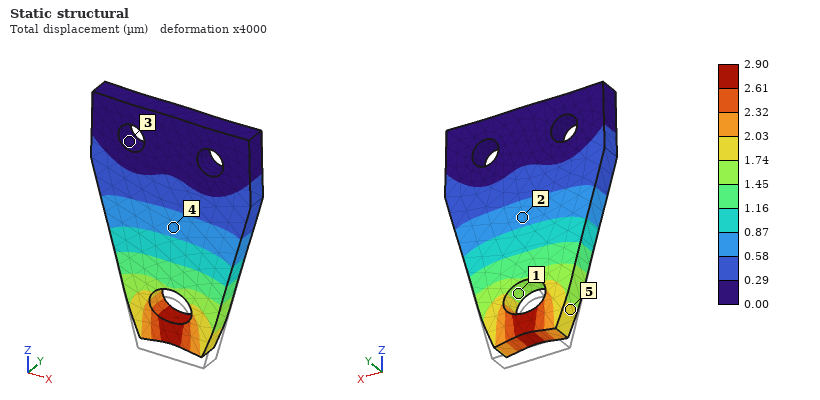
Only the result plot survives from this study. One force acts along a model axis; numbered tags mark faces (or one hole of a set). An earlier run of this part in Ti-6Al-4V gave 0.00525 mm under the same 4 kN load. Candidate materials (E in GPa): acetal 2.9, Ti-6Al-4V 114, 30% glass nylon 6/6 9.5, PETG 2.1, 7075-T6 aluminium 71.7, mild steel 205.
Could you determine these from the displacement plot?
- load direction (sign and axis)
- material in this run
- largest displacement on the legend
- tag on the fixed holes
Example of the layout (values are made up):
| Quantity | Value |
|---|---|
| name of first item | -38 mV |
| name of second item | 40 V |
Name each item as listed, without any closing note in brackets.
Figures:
| Quantity | Value |
|---|---|
| load direction | +Z |
| material in this run | mild steel |
| largest displacement on the legend | 2.90 µm |
| tag on the fixed holes | 3 |
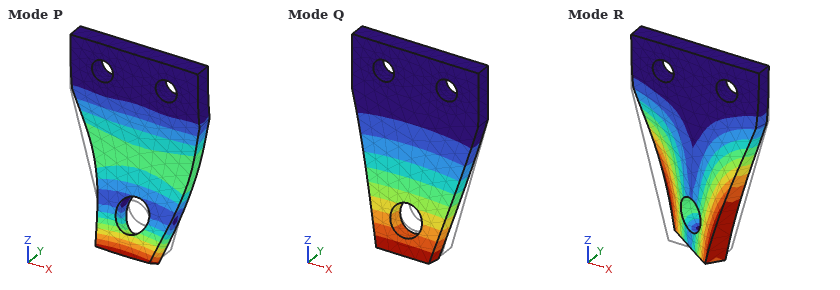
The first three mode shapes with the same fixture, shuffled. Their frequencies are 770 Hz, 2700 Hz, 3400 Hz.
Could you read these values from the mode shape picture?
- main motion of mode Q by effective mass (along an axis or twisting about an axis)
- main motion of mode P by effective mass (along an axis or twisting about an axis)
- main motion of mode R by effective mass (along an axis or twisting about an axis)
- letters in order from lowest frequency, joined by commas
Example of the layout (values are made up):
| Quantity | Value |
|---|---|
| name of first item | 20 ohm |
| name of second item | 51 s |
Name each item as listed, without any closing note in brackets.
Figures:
| Quantity | Value |
|---|---|
| main motion of mode Q by effective mass | along Y |
| main motion of mode P by effective mass | along Y |
| main motion of mode R by effective mass | twisting about Z |
| letters in order from lowest frequency, joined by commas | Q, R, P |
